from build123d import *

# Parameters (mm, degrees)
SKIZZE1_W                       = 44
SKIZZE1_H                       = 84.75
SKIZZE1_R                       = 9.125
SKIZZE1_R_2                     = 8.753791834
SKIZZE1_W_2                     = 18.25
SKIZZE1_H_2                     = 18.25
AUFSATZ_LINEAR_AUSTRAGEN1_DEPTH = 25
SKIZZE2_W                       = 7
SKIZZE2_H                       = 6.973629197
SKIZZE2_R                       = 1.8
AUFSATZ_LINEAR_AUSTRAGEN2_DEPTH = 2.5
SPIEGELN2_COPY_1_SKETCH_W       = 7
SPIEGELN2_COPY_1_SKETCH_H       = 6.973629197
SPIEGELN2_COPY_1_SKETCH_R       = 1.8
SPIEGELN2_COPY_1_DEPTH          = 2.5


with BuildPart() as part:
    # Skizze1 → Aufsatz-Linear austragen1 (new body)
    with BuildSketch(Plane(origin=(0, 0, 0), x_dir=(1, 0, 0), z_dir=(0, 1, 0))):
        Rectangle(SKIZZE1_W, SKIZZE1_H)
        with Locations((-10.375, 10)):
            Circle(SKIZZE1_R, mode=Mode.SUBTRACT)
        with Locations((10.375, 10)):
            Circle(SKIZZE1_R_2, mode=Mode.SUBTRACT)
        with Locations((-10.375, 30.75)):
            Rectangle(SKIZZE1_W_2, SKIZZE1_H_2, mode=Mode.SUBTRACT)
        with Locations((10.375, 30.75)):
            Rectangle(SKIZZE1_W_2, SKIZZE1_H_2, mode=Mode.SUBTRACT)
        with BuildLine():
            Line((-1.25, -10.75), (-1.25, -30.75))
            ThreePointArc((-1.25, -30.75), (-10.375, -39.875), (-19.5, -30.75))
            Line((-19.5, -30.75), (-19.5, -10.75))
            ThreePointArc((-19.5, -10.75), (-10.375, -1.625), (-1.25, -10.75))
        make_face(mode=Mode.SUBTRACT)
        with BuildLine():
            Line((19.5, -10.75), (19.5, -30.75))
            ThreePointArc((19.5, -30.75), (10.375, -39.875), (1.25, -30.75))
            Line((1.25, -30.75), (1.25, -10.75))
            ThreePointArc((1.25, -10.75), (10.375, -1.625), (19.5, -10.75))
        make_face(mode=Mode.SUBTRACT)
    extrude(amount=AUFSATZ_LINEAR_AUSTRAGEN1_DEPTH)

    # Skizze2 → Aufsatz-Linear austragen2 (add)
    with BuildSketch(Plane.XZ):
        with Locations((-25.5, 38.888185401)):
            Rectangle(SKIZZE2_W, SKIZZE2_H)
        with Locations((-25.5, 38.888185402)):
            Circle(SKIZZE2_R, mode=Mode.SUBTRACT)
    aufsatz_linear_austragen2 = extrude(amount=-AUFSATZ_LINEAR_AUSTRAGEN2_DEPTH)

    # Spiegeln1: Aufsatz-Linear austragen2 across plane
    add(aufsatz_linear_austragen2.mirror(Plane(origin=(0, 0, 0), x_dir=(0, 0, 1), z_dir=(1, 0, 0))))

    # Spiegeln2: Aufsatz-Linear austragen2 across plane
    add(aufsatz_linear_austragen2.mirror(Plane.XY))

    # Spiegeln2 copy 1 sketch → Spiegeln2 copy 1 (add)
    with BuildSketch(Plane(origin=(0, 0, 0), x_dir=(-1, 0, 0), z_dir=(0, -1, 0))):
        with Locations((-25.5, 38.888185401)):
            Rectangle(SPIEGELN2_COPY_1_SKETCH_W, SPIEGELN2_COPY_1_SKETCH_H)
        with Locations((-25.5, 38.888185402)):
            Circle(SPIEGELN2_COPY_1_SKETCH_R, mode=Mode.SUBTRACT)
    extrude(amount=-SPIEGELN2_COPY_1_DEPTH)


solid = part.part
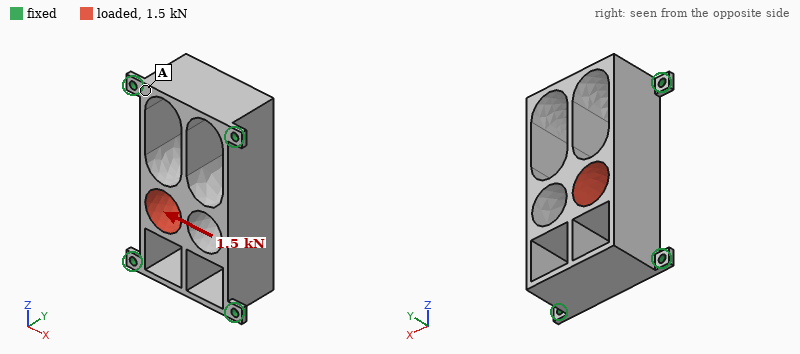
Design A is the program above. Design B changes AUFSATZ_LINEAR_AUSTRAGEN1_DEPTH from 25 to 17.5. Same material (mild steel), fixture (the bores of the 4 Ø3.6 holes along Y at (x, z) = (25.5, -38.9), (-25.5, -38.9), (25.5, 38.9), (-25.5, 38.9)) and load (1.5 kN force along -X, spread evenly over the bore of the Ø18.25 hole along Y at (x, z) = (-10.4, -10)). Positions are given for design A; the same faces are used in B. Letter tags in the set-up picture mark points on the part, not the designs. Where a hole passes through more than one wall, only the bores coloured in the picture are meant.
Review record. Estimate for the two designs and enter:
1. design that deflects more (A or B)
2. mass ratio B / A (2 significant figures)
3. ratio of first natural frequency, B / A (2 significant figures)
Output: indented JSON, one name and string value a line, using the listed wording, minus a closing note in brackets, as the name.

{
  "design that deflects more": "B",
  "mass ratio B / A": "0.70",
  "ratio of first natural frequency, B / A": "1.0"
}
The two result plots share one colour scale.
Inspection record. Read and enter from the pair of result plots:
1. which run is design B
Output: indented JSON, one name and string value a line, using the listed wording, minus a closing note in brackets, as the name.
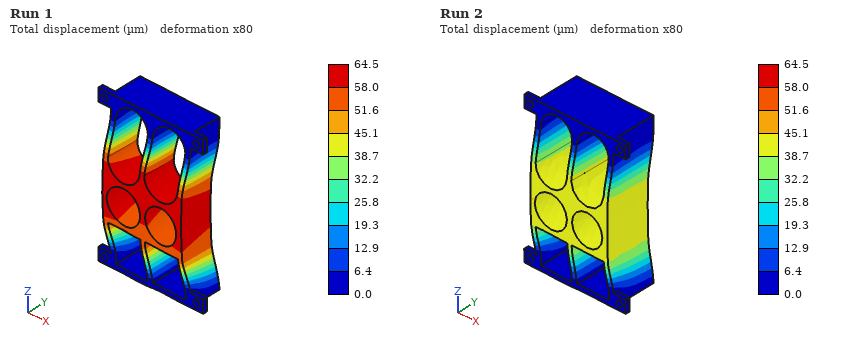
{
  "which run is design B": "Run 1"
}
